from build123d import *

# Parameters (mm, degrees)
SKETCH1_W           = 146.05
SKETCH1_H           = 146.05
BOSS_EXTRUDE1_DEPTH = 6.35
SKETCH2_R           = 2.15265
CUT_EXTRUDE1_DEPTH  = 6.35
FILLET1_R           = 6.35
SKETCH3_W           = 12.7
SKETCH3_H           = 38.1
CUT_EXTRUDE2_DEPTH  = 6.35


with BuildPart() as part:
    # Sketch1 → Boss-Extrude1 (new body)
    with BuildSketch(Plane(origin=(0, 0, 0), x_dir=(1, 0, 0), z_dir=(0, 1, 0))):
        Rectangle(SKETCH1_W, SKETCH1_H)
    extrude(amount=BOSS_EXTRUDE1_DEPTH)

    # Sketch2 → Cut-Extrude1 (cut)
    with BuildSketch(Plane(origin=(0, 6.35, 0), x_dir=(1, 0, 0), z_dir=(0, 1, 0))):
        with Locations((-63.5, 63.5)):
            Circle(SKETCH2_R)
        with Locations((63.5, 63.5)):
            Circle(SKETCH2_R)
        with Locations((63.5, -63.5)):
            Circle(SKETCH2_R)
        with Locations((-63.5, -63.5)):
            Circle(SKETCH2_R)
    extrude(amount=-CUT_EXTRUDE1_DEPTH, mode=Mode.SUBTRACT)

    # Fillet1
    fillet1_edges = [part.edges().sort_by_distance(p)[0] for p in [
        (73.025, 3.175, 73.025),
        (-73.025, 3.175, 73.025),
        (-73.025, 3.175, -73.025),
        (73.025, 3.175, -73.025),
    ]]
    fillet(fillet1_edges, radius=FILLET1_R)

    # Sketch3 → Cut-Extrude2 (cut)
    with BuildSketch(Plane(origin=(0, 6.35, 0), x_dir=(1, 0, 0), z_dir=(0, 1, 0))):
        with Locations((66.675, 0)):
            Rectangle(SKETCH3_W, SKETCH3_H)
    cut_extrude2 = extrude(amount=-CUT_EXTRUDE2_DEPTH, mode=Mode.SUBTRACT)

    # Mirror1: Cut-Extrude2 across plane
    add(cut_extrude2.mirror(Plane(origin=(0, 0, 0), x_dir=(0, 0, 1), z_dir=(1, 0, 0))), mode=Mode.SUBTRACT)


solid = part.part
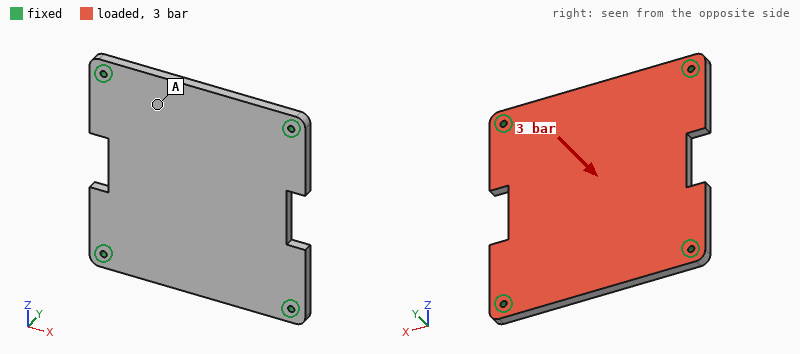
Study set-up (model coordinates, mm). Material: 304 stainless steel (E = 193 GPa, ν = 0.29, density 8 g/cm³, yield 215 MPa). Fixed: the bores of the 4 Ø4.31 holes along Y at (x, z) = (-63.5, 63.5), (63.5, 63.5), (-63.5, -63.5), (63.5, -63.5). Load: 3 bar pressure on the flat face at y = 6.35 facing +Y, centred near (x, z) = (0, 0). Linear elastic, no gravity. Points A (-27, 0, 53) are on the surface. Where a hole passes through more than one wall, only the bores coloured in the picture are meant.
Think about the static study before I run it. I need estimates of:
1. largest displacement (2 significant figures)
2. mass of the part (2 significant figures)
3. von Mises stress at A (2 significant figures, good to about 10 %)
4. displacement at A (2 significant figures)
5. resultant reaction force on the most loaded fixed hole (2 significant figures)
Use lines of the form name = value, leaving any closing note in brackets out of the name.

largest displacement = 0.16 mm
mass of the part = 1.0 kg
von Mises stress at A = 28 MPa
displacement at A = 0.082 mm
resultant reaction force on the most loaded fixed hole = 1.5 kN
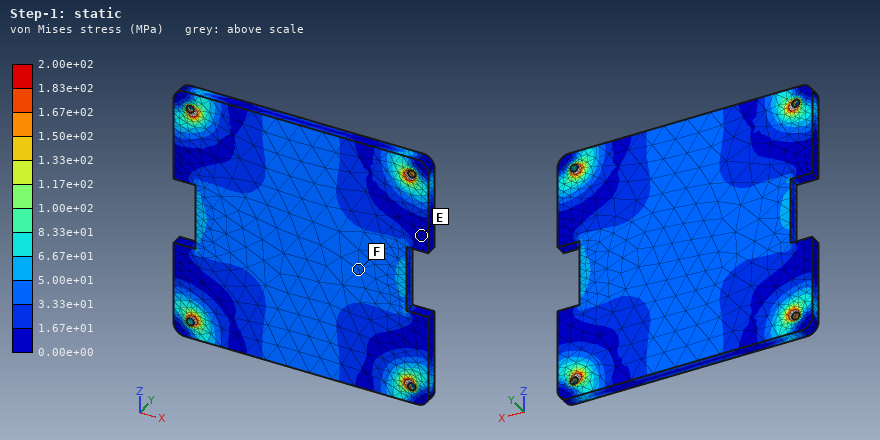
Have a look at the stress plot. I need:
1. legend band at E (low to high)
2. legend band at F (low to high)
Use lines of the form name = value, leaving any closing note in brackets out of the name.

legend band at E = 0.00e+00 to 1.67e+01 MPa
legend band at F = 3.33e+01 to 5.00e+01 MPa
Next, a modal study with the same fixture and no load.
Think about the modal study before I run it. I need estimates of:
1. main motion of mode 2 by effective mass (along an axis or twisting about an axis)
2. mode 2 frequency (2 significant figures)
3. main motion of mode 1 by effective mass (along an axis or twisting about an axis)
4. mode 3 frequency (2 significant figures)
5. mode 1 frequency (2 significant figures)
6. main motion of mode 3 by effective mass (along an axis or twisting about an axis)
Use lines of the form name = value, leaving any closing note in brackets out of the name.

main motion of mode 2 by effective mass = twisting about X
mode 2 frequency = 2000 Hz
main motion of mode 1 by effective mass = along Y
mode 3 frequency = 2200 Hz
mode 1 frequency = 1200 Hz
main motion of mode 3 by effective mass = twisting about Z
